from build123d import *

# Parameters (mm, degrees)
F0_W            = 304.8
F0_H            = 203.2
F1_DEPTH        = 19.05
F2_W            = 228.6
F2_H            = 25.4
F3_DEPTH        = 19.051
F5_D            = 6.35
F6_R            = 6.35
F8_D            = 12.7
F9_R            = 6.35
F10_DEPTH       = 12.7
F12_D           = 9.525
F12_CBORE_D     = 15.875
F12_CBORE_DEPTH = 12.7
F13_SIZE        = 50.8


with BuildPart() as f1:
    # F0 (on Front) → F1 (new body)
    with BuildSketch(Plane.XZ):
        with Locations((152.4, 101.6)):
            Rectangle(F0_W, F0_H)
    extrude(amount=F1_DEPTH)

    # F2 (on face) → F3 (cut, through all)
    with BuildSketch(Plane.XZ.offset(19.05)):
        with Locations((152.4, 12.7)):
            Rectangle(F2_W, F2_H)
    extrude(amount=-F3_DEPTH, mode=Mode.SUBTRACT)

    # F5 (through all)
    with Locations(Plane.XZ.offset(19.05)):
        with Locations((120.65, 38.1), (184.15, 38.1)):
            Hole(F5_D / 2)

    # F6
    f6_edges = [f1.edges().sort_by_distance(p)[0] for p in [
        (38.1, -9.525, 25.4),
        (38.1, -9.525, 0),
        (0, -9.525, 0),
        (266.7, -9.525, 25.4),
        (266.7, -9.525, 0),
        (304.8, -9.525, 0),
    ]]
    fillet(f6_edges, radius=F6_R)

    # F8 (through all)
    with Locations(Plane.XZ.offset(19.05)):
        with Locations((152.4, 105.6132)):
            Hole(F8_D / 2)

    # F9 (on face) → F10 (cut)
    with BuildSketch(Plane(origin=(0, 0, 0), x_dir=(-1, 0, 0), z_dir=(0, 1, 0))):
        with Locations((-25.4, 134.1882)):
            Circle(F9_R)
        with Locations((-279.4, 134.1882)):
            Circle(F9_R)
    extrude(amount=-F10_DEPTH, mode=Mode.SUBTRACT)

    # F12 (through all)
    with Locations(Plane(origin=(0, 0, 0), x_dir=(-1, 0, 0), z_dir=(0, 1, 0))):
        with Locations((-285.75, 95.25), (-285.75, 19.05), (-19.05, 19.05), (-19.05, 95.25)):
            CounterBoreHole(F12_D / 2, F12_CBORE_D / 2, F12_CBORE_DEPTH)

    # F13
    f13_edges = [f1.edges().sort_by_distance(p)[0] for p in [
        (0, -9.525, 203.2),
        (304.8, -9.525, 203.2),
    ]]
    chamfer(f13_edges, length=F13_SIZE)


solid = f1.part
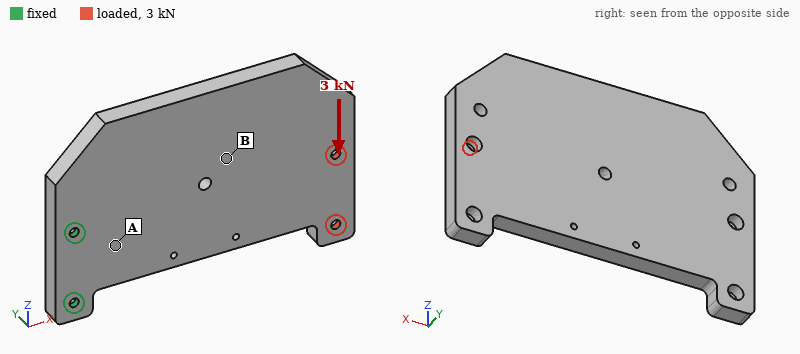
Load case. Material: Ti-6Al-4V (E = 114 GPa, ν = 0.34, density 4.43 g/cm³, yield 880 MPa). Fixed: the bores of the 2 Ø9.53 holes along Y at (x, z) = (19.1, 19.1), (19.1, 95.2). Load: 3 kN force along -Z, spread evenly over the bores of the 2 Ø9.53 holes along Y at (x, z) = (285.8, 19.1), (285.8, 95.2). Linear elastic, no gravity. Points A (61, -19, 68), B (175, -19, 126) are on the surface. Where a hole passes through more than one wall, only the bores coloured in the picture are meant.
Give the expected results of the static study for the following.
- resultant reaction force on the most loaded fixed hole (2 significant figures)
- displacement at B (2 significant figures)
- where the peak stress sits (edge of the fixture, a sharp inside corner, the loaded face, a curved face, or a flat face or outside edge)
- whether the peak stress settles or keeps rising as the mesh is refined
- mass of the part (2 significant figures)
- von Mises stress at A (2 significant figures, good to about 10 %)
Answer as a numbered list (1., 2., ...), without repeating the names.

1. 10 kN
2. 0.096 mm
3. edge of the fixture
4. keeps rising
5. 4.4 kg
6. 15 MPa
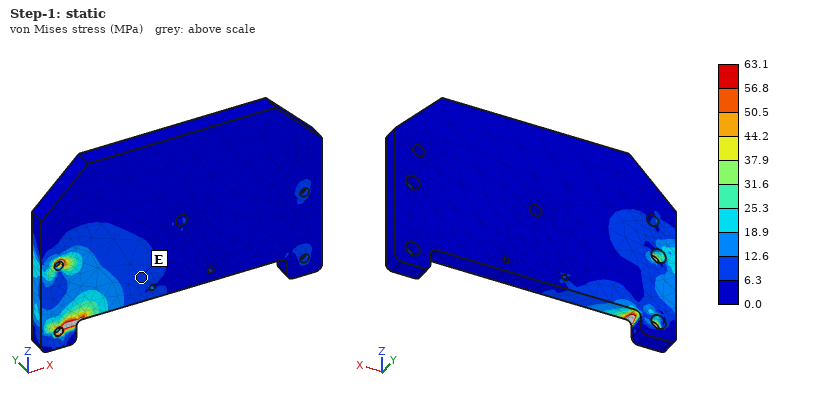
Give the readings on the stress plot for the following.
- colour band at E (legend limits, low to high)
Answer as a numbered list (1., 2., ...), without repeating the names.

1. 6.3 to 12.6 MPa
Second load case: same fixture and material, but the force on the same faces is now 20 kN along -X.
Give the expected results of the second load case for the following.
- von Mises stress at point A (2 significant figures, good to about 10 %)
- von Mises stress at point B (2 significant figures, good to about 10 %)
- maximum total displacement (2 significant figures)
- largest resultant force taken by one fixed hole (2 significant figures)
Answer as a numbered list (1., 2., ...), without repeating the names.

1. 23 MPa
2. 16 MPa
3. 0.54 mm
4. 10 kN
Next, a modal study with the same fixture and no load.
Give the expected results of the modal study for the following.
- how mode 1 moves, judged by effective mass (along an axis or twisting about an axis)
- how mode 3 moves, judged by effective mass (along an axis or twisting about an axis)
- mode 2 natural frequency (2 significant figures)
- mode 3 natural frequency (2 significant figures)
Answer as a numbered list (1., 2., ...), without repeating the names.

1. along Y
2. along Z
3. 460 Hz
4. 600 Hz
